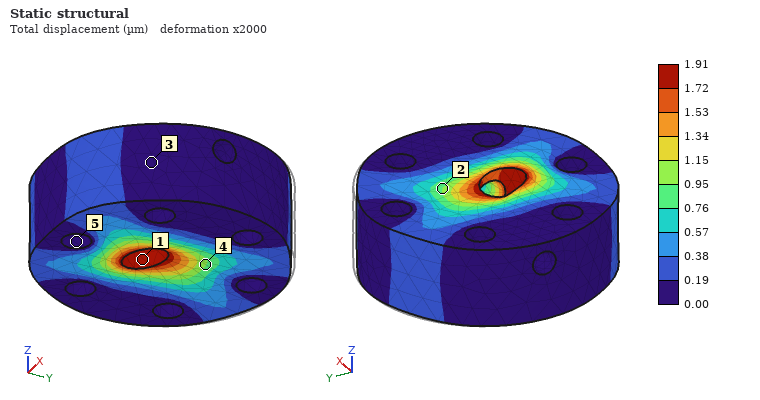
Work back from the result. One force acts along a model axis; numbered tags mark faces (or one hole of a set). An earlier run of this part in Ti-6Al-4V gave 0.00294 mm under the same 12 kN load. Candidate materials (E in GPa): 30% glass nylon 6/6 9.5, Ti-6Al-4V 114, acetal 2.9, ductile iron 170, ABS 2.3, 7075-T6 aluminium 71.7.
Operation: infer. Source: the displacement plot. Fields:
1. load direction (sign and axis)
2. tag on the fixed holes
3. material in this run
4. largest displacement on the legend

-Y
5
ductile iron
1.91 µm
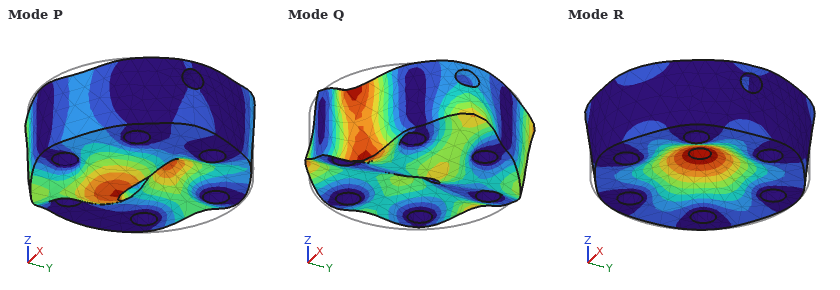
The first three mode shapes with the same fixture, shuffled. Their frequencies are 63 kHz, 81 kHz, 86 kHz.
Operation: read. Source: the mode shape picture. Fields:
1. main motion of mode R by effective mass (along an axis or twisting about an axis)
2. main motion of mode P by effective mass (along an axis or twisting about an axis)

along Z
twisting about X
